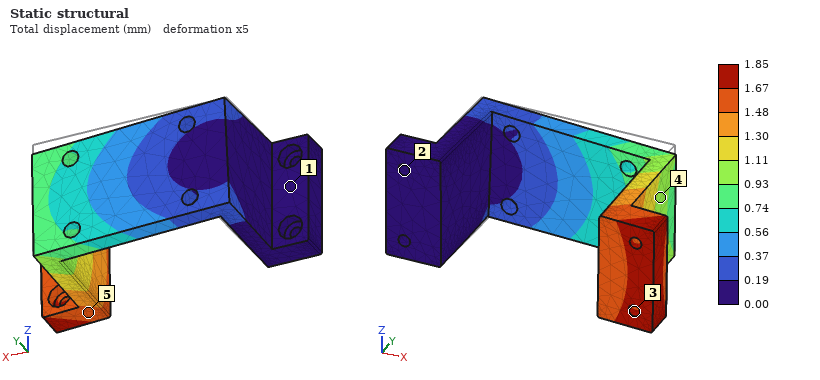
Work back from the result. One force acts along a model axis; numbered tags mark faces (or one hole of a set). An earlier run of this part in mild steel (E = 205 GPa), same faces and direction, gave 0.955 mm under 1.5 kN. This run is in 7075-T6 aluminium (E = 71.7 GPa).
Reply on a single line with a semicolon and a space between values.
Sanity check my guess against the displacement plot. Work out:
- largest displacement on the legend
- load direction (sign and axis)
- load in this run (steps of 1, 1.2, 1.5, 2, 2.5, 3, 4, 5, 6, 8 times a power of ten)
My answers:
1.85 mm; -Z; 1 kN
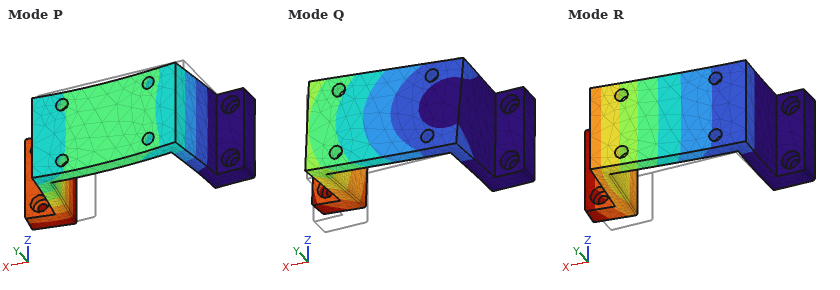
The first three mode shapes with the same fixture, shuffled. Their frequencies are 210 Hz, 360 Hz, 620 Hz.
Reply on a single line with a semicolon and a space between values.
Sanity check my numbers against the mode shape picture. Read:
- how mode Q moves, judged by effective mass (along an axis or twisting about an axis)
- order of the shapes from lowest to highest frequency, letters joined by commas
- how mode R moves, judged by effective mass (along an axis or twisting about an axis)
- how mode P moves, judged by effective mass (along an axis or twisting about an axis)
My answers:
along Z; R, Q, P; along Y; along X
